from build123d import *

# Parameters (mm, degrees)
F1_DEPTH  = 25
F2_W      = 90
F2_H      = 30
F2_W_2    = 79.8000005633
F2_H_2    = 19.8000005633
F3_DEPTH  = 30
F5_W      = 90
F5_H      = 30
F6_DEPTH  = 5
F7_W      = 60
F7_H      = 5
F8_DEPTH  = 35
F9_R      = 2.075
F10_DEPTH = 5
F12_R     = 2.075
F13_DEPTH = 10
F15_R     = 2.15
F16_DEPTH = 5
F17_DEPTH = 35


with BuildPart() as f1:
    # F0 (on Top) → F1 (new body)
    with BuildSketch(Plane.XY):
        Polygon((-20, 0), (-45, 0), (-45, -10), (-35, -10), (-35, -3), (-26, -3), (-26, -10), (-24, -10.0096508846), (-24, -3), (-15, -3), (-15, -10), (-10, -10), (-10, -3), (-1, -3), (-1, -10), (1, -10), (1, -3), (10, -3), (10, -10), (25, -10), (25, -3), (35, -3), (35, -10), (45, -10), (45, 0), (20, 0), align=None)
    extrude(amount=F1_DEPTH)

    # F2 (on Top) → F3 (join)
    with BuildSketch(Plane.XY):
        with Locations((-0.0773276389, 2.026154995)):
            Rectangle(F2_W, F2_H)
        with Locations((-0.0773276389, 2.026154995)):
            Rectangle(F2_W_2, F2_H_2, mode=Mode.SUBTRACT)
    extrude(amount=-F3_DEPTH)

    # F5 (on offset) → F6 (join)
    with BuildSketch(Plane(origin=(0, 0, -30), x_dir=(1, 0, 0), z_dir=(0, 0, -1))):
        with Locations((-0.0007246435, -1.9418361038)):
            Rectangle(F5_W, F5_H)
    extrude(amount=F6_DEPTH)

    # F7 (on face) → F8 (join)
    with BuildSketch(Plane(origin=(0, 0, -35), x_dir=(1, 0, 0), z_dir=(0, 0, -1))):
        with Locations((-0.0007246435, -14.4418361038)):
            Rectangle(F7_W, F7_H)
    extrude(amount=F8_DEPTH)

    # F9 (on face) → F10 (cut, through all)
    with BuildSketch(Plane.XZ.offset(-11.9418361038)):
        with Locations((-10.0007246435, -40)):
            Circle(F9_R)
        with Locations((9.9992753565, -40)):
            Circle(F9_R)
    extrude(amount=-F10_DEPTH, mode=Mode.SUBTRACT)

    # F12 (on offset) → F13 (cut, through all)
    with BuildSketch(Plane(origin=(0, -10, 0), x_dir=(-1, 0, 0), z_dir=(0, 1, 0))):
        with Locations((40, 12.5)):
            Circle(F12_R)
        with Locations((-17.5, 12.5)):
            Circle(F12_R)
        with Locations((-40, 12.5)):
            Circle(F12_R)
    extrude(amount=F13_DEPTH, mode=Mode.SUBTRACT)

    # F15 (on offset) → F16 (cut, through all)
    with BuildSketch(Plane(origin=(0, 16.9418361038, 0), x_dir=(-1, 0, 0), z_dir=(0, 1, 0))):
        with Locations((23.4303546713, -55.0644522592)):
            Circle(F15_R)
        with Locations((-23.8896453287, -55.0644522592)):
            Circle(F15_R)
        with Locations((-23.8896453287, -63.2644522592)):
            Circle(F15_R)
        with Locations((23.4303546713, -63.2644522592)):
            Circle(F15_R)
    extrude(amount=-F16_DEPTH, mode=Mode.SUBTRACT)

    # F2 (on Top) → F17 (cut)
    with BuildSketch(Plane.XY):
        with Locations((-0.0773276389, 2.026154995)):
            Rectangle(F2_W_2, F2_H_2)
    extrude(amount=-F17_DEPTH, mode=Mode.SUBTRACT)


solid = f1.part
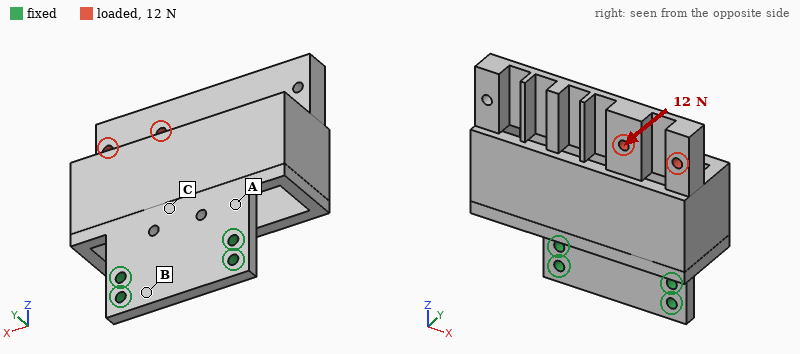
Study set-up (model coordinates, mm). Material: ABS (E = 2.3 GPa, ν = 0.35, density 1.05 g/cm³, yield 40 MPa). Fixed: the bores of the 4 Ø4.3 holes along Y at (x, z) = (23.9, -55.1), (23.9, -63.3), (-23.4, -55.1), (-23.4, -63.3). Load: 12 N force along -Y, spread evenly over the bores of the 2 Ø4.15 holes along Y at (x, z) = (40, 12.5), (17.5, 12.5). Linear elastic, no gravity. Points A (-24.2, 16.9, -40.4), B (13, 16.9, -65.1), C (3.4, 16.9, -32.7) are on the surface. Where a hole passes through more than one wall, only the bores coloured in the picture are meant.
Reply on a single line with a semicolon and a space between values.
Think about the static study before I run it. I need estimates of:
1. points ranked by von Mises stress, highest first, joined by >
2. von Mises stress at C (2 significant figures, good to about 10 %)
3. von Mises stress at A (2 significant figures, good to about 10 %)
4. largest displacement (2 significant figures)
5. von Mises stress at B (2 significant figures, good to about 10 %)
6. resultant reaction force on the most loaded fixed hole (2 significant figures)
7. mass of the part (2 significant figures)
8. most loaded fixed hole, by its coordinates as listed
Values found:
A > C > B; 1.8 MPa; 2.8 MPa; 1.3 mm; 0.80 MPa; 31 N; 66 g; (23.9, -55.1)
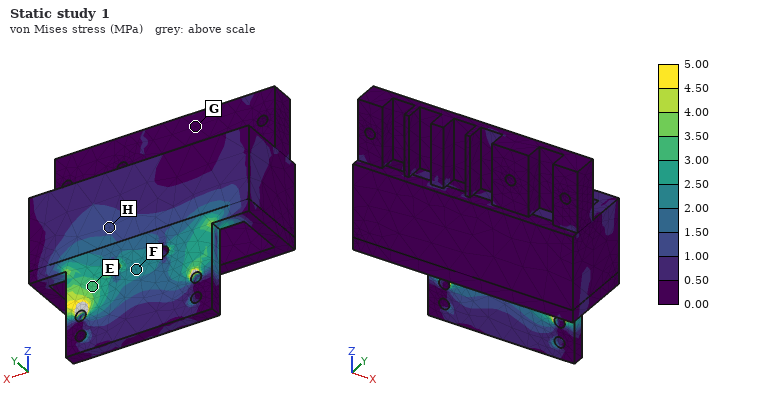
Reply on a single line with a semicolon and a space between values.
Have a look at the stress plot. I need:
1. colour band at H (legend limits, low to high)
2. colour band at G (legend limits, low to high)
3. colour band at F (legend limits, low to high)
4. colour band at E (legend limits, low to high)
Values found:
1.00 to 1.50 MPa; 0.00 to 0.50 MPa; 2.00 to 2.50 MPa; 3.00 to 3.50 MPa
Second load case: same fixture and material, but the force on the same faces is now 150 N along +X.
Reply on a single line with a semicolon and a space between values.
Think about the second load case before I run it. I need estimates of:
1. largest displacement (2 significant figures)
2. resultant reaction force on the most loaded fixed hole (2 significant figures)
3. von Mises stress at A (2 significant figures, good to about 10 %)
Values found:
1.3 mm; 200 N; 7.3 MPa
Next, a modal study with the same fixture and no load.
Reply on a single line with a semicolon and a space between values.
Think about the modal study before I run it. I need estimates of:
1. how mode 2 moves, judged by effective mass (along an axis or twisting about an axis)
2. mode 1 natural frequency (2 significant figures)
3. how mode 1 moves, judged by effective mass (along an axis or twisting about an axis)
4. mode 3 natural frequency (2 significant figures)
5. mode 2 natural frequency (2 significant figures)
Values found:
along X; 110 Hz; along Y; 480 Hz; 230 Hz
